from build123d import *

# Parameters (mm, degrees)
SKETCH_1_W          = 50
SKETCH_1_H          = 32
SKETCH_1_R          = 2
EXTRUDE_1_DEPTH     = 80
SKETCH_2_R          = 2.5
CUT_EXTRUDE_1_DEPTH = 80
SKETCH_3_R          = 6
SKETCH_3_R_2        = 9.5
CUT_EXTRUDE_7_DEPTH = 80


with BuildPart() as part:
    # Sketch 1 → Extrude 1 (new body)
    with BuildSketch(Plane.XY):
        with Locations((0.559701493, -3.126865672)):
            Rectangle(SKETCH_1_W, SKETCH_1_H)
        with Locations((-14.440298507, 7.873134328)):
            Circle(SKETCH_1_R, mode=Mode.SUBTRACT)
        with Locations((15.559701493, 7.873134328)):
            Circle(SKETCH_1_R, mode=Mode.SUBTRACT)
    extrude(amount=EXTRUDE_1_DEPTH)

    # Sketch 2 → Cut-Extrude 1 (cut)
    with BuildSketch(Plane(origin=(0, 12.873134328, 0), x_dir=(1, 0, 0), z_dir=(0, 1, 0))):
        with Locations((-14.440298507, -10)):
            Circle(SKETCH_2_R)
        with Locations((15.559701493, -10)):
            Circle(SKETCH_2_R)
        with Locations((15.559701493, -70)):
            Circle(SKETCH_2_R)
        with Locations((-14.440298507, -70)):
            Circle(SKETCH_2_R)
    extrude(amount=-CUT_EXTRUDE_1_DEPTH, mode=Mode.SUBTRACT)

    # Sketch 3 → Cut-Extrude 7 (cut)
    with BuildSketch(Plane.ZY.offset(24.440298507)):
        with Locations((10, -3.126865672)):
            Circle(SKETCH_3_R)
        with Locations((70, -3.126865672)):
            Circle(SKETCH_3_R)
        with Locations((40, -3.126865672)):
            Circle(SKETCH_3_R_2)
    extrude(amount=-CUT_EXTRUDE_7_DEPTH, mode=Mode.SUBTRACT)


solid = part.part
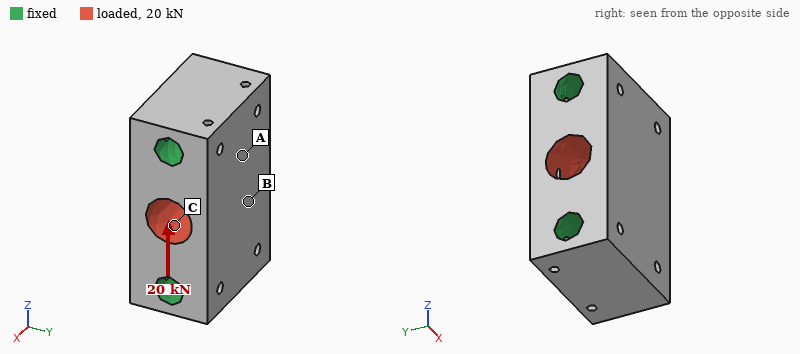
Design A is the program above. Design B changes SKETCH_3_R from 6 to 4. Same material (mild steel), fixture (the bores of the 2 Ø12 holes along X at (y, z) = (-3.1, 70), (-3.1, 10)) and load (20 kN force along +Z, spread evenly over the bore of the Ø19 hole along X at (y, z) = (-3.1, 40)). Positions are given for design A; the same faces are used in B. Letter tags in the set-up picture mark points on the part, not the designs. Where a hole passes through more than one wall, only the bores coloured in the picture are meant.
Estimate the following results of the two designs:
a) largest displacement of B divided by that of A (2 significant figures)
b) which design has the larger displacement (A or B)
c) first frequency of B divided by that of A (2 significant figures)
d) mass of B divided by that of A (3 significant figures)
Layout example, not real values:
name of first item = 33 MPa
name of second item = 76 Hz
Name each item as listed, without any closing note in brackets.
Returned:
largest displacement of B divided by that of A = 1.1
which design has the larger displacement = B
first frequency of B divided by that of A = 0.83
mass of B divided by that of A = 1.06
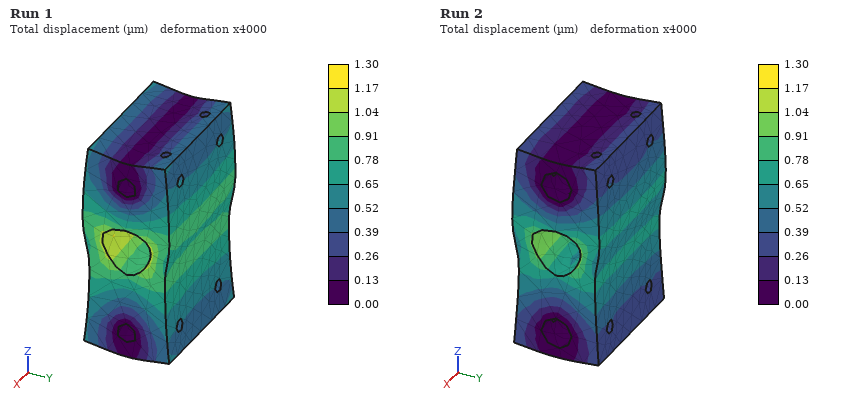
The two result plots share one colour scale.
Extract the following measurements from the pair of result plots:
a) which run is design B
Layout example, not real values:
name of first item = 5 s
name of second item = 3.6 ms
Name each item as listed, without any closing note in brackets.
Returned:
which run is design B = Run 1
